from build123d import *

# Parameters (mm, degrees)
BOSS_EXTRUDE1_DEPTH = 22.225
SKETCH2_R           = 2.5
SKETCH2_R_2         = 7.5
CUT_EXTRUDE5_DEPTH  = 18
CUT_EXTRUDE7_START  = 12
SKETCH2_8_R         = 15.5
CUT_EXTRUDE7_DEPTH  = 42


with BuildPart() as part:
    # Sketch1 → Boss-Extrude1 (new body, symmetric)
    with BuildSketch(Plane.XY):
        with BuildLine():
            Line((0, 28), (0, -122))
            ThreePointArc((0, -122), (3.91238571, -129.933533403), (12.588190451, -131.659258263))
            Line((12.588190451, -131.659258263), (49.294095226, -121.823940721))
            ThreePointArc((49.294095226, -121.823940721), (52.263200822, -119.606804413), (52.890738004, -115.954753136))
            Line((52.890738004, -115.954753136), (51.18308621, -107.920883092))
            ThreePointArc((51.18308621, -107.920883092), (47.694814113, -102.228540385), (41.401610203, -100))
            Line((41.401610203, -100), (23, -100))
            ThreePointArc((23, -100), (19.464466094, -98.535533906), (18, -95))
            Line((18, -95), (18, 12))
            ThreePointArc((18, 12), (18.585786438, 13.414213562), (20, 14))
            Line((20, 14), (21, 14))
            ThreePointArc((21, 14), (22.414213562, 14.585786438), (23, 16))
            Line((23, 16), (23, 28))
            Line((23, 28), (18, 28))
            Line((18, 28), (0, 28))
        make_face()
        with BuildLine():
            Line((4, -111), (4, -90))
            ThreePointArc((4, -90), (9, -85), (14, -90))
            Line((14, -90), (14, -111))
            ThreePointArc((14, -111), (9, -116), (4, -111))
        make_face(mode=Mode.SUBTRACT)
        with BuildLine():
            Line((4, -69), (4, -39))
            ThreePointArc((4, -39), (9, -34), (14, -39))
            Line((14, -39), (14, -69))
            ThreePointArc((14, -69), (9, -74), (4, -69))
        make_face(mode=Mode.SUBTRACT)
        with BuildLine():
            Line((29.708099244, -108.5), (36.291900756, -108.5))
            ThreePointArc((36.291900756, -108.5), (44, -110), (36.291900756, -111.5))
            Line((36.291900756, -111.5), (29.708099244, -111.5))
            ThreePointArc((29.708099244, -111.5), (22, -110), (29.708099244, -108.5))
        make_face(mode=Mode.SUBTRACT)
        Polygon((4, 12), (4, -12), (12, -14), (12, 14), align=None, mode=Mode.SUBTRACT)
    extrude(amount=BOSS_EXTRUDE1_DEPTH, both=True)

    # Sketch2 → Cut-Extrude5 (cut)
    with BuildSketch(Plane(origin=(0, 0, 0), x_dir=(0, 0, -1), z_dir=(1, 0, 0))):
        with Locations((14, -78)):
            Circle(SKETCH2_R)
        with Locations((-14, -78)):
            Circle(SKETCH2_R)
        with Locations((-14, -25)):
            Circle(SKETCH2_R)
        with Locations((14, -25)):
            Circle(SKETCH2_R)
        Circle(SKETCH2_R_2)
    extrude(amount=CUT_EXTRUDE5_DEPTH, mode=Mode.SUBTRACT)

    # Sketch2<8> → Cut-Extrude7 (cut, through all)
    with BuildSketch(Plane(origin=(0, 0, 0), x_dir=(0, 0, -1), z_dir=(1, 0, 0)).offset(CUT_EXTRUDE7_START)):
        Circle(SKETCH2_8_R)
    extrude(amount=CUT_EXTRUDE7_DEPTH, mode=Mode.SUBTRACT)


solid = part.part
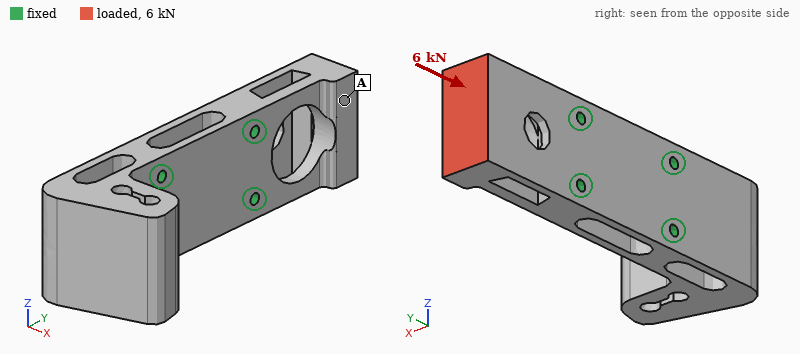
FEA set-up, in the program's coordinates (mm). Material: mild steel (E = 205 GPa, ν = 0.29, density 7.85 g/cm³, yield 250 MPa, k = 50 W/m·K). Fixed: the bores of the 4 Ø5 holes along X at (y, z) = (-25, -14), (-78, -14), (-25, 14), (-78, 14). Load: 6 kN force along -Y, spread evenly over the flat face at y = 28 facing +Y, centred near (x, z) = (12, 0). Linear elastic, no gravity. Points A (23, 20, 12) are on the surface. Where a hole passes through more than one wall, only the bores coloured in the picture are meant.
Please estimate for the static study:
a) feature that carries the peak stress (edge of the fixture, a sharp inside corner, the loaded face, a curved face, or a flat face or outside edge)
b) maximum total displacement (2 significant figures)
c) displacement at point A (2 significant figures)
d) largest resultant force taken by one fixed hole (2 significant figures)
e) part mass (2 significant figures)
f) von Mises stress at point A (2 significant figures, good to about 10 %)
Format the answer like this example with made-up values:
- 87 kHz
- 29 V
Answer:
- a curved face
- 24 µm
- 19 µm
- 2.9 kN
- 920 g
- 12 MPa
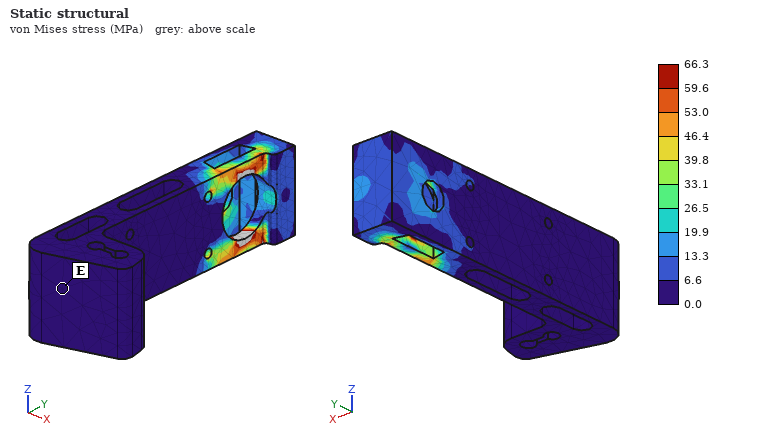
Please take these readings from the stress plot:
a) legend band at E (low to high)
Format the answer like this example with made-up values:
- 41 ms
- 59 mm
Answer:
- 0.0 to 6.6 MPa
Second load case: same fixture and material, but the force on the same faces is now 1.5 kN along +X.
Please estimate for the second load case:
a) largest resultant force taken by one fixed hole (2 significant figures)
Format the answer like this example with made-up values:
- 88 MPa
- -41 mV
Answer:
- 790 N
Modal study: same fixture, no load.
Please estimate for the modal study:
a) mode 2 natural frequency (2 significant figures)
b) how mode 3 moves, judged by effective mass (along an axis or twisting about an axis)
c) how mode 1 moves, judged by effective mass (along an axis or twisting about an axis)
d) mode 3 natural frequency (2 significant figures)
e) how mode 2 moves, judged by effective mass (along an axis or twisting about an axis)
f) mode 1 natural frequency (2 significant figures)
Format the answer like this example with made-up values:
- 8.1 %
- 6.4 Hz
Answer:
- 2400 Hz
- along Z
- along X
- 2700 Hz
- along X
- 1800 Hz
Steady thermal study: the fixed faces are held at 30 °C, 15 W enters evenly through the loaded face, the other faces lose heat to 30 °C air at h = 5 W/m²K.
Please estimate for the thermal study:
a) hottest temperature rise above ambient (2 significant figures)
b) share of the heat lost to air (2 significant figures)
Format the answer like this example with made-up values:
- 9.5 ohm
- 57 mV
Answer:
- 44 K
- 6.7 %
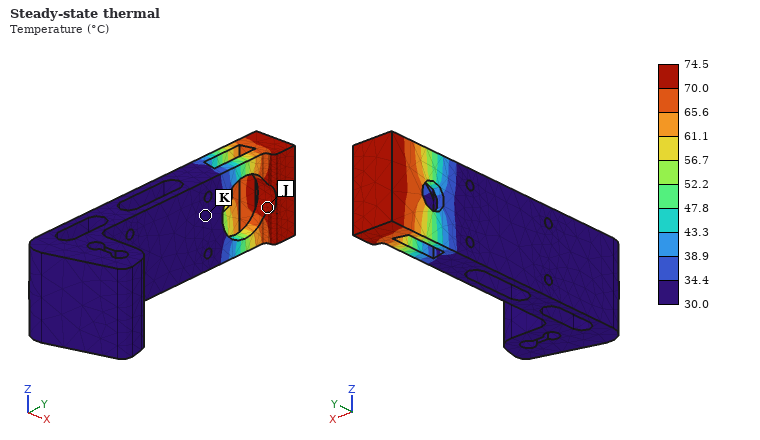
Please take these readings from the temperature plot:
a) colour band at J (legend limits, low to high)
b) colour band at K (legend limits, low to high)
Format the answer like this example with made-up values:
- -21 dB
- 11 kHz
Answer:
- 70.0 to 74.5 °C
- 30.0 to 34.4 °C
